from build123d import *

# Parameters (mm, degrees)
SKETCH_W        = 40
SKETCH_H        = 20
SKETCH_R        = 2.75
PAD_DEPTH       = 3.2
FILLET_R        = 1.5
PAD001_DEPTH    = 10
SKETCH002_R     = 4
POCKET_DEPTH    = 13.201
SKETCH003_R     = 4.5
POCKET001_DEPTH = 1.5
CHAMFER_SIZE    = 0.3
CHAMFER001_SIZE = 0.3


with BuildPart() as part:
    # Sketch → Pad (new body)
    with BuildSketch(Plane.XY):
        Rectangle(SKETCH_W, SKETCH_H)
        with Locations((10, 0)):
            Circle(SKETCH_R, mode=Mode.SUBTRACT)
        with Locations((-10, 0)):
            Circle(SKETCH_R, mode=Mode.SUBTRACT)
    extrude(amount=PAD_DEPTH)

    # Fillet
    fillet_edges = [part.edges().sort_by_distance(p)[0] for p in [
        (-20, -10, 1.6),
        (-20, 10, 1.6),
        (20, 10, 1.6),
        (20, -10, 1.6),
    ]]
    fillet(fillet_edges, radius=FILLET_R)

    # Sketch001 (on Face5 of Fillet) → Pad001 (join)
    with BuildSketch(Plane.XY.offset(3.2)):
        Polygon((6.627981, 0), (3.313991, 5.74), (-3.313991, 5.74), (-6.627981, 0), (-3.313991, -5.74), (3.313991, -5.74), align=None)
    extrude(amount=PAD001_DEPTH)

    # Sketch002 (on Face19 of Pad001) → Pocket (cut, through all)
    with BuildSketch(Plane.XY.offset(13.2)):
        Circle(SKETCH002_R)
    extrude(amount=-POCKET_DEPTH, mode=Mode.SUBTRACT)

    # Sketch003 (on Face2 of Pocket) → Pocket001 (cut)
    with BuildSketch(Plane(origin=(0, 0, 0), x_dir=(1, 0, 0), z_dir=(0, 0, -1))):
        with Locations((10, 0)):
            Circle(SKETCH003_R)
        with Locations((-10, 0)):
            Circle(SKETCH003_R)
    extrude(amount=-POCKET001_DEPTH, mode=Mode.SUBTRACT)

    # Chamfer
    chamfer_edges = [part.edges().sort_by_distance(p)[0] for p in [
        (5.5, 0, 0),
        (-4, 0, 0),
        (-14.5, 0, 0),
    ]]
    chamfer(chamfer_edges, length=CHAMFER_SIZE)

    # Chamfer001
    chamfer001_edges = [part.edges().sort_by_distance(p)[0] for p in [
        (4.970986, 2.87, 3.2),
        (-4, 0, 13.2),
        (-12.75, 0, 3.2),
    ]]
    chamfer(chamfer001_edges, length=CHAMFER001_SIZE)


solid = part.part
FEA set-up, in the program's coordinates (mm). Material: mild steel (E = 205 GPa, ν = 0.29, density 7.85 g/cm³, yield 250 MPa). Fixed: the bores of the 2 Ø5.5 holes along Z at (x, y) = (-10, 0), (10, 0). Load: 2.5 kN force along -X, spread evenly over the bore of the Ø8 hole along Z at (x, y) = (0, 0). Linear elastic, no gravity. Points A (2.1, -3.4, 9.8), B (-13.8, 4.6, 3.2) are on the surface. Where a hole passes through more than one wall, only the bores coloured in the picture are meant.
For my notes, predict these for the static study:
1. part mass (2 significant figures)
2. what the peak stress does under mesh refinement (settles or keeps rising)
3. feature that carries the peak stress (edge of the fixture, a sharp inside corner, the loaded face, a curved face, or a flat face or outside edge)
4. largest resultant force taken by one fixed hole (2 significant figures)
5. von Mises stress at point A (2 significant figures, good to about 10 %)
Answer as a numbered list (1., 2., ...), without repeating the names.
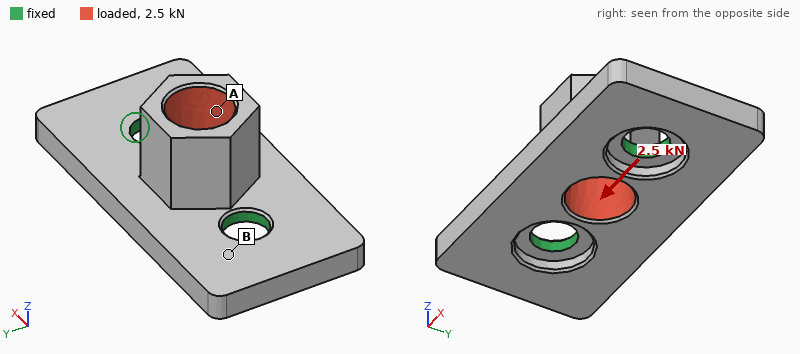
1. 22 g
2. keeps rising
3. a sharp inside corner
4. 1.5 kN
5. 40 MPa
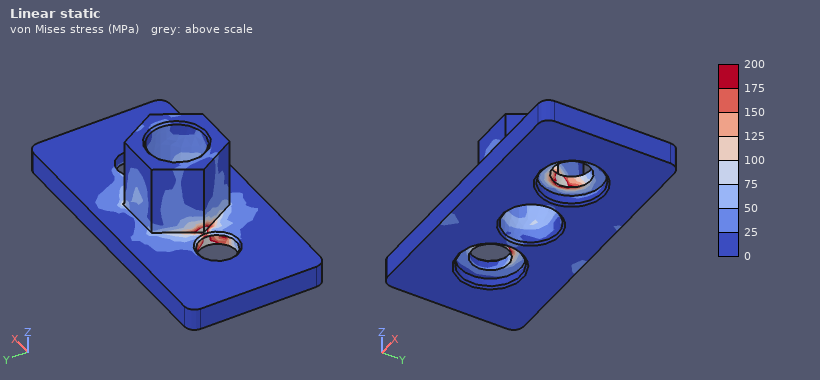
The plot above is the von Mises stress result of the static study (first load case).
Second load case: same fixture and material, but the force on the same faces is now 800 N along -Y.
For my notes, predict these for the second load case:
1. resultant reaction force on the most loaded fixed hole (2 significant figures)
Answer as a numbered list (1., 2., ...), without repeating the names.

1. 410 N
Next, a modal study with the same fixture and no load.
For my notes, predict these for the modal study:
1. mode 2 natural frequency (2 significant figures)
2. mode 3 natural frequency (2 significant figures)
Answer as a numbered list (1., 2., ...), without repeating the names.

1. 18 kHz
2. 18 kHz
